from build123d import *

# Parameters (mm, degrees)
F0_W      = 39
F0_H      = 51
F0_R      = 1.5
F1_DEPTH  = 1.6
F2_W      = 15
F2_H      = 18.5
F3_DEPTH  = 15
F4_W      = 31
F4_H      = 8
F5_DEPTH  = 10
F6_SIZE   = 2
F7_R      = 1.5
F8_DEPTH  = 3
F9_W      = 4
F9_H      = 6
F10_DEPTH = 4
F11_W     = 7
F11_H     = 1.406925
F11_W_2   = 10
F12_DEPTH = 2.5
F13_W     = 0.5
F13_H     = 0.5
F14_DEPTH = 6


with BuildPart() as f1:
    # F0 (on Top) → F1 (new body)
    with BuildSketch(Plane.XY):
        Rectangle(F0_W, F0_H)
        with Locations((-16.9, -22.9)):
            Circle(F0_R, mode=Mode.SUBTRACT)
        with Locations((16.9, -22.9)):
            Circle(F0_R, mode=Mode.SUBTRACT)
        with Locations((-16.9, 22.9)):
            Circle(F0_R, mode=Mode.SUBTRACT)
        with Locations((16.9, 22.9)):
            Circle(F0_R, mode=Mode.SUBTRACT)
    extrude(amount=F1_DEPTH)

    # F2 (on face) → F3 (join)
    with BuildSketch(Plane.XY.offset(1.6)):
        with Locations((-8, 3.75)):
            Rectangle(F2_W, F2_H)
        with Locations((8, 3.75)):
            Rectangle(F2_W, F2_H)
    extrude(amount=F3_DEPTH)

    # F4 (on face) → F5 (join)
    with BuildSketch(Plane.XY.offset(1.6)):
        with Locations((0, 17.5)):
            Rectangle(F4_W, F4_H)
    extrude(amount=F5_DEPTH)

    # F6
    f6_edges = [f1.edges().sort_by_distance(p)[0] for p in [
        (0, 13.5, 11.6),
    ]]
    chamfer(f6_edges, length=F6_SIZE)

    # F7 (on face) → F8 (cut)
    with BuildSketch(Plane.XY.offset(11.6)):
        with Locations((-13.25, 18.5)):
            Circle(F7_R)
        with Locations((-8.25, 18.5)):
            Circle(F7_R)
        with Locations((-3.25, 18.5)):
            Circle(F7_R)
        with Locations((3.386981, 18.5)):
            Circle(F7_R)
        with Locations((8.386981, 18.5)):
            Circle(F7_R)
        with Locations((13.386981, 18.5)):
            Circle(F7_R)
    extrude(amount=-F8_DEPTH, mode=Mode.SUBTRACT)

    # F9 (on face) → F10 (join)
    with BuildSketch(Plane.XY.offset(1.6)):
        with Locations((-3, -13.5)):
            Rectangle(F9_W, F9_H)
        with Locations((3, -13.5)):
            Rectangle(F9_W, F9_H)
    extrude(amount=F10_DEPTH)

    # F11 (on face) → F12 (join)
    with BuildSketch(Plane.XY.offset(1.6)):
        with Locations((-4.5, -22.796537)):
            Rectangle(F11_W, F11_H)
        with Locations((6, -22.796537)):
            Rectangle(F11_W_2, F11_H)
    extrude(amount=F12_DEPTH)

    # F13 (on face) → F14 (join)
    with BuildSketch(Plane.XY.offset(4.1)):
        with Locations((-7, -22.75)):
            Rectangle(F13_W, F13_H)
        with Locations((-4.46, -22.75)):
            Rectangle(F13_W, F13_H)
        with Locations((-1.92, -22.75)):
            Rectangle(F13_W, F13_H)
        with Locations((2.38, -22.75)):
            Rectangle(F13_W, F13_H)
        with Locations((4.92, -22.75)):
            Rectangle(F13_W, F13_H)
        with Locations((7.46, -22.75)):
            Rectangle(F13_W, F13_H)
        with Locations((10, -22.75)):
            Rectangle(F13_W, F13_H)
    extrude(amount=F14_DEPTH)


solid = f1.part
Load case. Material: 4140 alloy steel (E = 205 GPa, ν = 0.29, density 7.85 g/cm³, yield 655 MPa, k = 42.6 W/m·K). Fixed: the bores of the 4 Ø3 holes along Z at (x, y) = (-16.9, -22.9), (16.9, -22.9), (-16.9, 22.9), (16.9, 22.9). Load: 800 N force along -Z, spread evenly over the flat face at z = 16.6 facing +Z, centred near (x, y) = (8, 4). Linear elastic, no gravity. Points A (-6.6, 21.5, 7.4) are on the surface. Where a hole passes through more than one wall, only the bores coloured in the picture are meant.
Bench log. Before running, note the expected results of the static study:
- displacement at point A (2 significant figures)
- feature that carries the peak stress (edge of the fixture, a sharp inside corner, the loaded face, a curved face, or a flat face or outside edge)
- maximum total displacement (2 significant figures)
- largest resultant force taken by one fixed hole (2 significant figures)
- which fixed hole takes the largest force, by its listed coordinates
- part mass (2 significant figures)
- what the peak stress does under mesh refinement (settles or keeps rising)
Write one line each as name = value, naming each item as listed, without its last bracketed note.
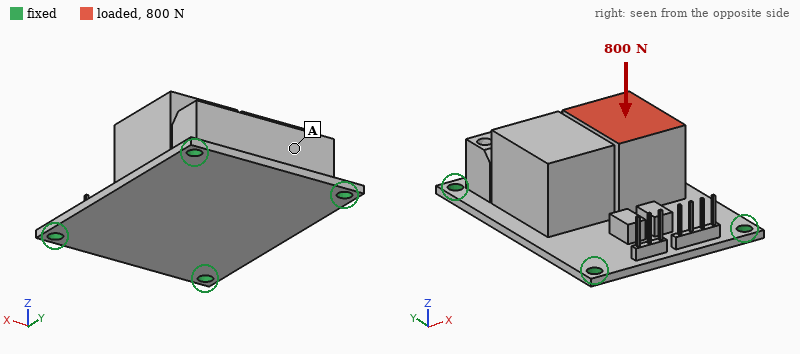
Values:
displacement at point A = 20 µm
feature that carries the peak stress = edge of the fixture
maximum total displacement = 76 µm
largest resultant force taken by one fixed hole = 490 N
which fixed hole takes the largest force, by its listed coordinates = (16.9, 22.9)
part mass = 110 g
what the peak stress does under mesh refinement = keeps rising
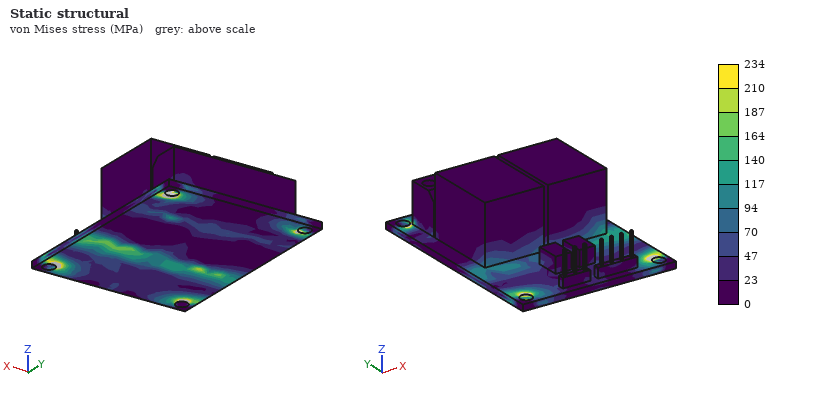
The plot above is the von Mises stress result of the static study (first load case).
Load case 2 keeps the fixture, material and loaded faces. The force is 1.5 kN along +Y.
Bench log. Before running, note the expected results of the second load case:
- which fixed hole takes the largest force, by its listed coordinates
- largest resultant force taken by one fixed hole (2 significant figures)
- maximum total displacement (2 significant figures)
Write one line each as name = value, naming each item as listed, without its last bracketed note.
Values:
which fixed hole takes the largest force, by its listed coordinates = (16.9, 22.9)
largest resultant force taken by one fixed hole = 680 N
maximum total displacement = 0.14 mm
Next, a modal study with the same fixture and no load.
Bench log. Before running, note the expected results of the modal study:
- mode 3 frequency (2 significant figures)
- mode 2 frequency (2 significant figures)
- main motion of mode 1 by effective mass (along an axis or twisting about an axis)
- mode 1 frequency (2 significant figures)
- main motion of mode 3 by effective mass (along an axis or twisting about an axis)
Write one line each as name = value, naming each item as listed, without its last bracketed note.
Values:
mode 3 frequency = 5400 Hz
mode 2 frequency = 4700 Hz
main motion of mode 1 by effective mass = along Z
mode 1 frequency = 2000 Hz
main motion of mode 3 by effective mass = along X
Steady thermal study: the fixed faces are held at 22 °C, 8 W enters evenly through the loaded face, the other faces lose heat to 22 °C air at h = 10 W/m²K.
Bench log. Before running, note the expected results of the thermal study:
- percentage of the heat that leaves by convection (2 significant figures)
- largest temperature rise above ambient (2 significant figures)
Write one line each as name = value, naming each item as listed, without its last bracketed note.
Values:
percentage of the heat that leaves by convection = 17 %
largest temperature rise above ambient = 38 K
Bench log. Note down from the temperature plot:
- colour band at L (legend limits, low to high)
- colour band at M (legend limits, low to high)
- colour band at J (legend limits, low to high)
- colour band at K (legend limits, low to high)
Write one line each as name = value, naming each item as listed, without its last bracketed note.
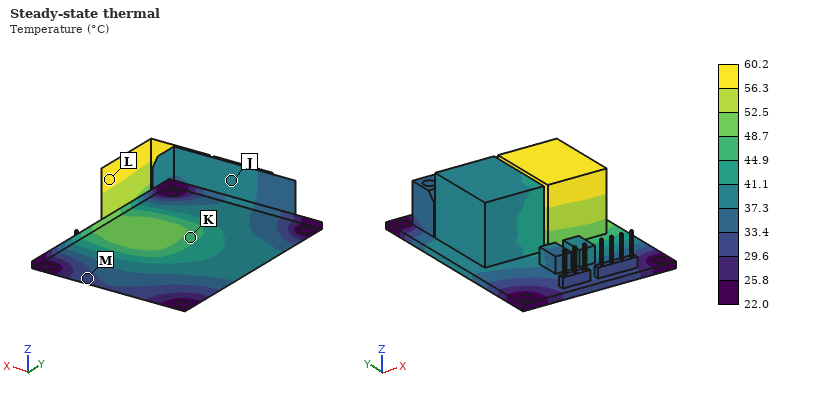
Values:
colour band at L = 56.3 to 60.2 °C
colour band at M = 29.6 to 33.4 °C
colour band at J = 37.3 to 41.1 °C
colour band at K = 44.9 to 48.7 °C
